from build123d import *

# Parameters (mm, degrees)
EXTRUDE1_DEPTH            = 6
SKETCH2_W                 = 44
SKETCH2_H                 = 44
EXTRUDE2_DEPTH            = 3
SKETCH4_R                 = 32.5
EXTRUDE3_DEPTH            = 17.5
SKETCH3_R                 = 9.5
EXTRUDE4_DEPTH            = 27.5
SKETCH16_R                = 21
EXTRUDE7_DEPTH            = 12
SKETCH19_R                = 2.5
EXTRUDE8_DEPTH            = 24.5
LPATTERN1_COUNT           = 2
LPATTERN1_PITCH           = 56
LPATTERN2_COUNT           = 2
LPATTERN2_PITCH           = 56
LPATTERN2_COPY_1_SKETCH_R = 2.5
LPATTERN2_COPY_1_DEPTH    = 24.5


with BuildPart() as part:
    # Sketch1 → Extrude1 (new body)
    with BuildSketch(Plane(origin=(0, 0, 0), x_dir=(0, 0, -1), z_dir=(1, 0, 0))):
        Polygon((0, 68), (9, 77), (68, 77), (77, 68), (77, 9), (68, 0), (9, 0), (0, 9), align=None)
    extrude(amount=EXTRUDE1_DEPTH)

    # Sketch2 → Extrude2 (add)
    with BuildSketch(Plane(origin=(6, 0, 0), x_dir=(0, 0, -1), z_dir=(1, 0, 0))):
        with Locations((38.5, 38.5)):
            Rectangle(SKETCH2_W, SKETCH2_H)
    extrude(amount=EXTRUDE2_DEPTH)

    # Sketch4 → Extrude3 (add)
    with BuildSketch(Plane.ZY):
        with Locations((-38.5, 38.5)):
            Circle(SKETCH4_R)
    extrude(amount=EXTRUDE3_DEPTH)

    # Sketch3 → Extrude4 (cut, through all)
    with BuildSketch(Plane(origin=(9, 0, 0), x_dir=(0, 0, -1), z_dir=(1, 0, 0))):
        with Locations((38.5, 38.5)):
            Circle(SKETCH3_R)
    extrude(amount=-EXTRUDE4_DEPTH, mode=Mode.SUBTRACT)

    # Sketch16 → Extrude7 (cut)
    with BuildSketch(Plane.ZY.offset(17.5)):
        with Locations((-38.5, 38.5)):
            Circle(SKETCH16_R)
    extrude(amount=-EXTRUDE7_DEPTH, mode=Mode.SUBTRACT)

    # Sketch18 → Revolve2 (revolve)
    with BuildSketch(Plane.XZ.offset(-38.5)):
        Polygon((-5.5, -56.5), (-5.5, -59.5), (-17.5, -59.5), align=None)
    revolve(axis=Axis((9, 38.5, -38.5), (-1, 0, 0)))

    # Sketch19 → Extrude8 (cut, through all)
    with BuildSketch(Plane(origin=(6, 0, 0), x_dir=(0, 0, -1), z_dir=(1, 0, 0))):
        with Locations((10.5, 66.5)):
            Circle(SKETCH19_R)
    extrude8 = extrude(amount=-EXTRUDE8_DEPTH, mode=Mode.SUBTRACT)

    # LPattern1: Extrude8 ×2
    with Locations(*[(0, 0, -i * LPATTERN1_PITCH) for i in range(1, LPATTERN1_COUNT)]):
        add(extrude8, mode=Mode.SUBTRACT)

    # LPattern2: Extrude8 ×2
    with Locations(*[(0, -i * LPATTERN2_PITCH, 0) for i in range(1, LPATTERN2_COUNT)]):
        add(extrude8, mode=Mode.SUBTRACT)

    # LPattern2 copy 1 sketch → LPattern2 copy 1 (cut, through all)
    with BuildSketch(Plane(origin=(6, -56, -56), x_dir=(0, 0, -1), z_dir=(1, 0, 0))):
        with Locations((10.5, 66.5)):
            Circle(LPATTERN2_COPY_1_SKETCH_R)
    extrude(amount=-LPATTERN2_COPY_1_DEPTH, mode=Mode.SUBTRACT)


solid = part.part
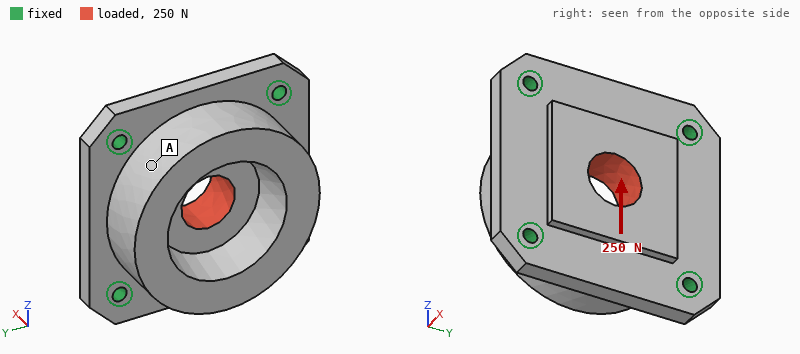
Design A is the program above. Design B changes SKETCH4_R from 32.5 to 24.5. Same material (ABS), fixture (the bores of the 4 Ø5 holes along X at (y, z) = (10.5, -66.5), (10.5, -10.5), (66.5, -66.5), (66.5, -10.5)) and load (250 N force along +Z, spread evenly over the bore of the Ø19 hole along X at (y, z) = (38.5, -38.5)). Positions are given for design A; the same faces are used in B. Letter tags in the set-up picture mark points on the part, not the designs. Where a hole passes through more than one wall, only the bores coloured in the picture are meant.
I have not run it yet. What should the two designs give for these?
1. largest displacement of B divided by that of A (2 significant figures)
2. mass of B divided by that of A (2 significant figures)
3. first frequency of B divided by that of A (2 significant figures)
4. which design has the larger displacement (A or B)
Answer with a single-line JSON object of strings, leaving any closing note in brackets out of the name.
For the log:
{"largest displacement of B divided by that of A": "1.2", "mass of B divided by that of A": "0.68", "first frequency of B divided by that of A": "0.85", "which design has the larger displacement": "B"}
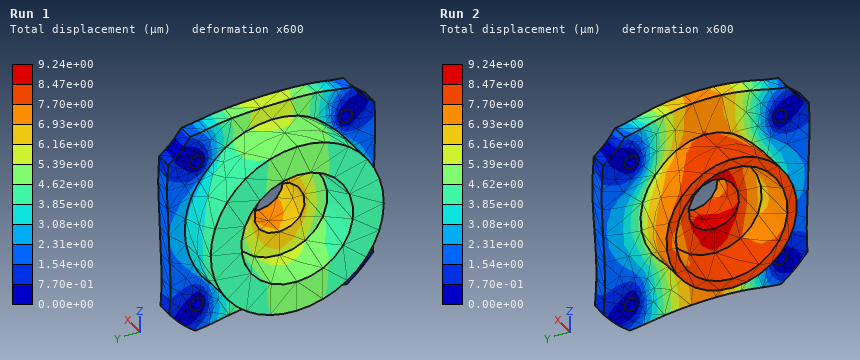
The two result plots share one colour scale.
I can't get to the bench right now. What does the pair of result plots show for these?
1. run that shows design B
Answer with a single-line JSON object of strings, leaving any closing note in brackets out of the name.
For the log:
{"run that shows design B": "Run 2"}
